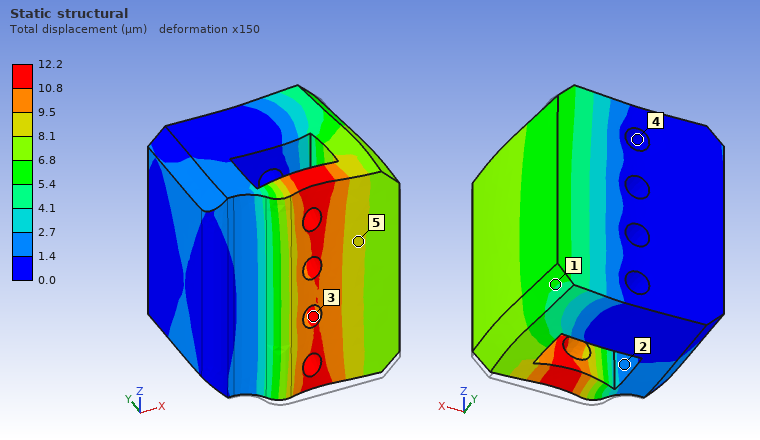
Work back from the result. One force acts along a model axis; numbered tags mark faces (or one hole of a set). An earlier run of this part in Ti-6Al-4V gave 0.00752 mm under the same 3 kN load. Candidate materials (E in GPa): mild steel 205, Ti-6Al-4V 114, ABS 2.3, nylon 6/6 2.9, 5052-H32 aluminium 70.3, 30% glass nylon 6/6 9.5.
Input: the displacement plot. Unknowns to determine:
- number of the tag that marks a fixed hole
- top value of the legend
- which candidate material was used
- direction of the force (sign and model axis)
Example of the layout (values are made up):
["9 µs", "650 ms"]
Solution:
["4", "12.2 µm", "5052-H32 aluminium", "+Y"]
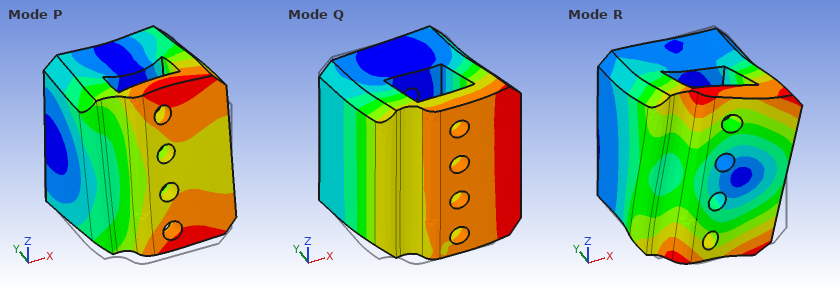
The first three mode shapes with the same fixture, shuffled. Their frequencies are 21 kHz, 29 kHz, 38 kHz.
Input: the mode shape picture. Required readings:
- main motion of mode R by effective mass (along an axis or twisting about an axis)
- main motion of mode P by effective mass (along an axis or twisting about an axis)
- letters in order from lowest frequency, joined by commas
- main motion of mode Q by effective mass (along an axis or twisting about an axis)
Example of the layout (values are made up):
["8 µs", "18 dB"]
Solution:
["twisting about Y", "along Z", "Q, P, R", "along X"]
